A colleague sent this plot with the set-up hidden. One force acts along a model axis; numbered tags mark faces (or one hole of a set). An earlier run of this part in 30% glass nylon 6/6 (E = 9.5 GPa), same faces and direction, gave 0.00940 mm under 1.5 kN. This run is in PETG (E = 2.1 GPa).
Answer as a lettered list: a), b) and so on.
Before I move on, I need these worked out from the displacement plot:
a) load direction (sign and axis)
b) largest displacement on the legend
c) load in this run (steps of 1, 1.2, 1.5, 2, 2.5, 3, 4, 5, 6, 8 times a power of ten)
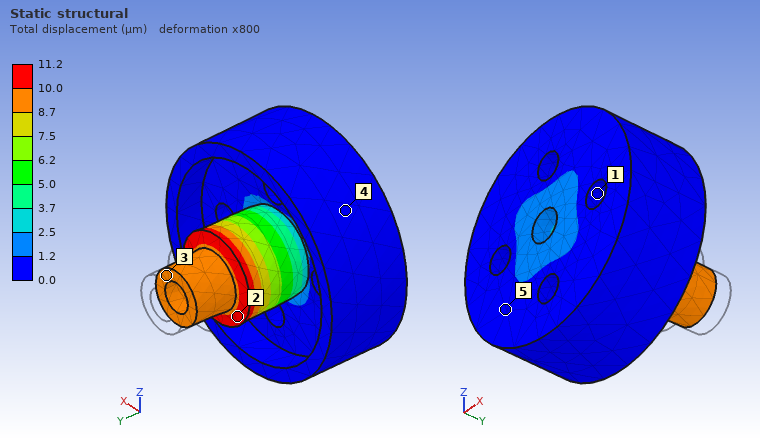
a) -Y
b) 11.2 µm
c) 400 N
